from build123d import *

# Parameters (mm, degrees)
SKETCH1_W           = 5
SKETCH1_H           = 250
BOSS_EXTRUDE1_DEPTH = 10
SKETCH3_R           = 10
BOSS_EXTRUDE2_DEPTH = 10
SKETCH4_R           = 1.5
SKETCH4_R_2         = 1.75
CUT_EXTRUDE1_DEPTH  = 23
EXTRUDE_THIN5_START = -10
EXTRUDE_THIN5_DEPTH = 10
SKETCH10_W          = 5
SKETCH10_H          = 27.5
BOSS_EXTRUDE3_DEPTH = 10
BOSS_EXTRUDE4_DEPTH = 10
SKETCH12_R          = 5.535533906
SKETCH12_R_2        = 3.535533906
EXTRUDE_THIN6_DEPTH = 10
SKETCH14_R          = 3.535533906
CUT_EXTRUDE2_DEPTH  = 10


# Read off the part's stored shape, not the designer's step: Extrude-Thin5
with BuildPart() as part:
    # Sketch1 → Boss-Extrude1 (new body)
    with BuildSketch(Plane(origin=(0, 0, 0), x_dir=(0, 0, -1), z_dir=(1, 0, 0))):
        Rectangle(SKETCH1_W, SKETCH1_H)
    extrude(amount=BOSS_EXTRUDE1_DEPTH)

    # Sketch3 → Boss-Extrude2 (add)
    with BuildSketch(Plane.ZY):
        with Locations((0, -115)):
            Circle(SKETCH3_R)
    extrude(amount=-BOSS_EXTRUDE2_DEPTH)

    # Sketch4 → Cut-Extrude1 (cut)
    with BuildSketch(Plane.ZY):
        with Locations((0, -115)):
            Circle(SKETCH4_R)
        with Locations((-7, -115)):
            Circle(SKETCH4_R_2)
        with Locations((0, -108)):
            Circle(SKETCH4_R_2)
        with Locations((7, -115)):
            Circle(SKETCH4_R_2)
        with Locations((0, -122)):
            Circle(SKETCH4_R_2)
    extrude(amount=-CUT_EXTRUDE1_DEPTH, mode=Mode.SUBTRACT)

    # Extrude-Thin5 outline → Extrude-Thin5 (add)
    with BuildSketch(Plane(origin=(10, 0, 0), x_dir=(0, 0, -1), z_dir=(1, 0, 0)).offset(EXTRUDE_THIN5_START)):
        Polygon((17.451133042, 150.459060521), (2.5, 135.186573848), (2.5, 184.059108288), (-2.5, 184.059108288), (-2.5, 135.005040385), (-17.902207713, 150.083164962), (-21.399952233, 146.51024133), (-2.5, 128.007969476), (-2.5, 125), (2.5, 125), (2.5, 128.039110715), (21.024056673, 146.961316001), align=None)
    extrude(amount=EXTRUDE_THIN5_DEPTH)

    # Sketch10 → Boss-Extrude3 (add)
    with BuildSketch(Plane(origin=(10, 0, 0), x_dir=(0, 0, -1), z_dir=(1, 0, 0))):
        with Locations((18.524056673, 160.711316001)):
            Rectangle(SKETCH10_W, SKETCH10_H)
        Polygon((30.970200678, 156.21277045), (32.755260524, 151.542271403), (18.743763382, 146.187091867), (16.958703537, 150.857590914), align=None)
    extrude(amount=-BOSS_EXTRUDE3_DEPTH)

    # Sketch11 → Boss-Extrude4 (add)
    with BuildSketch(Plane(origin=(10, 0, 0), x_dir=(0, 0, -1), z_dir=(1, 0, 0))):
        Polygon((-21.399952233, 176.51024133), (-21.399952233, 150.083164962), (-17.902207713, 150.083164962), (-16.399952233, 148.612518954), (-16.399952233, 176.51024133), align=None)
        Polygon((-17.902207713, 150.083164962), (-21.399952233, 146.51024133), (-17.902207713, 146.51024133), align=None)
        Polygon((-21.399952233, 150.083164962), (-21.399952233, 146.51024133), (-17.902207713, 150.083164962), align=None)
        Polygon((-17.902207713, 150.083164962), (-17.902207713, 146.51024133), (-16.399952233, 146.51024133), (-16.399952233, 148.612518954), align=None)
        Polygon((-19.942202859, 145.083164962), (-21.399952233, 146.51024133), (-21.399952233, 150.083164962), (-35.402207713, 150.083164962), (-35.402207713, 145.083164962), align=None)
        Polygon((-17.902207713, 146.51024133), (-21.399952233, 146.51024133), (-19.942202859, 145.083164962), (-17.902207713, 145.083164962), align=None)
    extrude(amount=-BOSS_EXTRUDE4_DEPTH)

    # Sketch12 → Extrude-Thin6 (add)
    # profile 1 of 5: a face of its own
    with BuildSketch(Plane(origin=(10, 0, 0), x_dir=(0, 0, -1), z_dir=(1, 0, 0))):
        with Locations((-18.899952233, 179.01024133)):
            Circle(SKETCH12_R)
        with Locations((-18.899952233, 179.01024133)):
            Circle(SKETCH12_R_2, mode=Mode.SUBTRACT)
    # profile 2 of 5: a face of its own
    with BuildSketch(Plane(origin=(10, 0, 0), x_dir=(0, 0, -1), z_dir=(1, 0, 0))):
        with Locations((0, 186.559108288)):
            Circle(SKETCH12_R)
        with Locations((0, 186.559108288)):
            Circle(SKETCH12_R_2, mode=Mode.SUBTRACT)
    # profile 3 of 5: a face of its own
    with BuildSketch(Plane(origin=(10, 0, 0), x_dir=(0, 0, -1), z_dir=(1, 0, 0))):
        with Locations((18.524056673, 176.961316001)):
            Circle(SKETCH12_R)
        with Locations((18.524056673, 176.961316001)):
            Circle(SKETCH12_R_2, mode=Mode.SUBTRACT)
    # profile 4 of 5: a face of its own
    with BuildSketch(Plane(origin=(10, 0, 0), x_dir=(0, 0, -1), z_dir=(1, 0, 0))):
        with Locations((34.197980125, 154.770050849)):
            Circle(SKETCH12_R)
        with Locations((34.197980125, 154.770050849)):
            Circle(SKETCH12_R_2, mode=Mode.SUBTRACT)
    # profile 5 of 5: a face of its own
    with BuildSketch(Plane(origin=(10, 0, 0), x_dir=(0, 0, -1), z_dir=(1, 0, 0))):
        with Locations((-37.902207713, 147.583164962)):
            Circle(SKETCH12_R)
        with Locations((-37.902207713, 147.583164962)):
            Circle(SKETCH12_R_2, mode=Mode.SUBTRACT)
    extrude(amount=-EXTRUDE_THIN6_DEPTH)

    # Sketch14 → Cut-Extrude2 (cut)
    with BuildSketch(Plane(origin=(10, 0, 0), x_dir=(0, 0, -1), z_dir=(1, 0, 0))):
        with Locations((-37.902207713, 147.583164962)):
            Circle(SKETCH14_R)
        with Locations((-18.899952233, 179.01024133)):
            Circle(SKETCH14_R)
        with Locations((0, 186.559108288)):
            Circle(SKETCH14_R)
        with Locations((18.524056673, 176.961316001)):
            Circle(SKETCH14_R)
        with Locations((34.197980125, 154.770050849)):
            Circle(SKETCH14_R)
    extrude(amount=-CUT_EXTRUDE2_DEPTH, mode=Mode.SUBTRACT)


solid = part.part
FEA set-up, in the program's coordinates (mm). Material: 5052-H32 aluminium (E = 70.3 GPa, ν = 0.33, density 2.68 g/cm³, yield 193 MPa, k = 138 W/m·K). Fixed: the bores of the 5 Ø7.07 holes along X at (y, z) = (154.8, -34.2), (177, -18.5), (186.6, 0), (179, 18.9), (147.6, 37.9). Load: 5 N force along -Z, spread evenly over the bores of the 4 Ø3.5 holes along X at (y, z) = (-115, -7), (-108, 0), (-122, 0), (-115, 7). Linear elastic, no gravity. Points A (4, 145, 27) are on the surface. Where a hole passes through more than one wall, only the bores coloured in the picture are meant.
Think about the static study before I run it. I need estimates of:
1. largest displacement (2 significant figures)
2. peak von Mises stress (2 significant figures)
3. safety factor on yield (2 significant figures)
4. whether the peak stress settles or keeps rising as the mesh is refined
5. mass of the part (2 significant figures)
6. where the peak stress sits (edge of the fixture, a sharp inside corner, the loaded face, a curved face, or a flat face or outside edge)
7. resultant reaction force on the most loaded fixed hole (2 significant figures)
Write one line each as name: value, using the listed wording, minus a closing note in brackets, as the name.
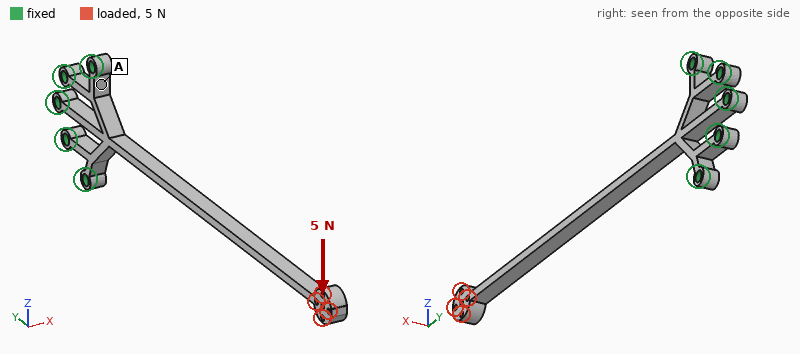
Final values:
largest displacement: 3.6 mm
peak von Mises stress: 28 MPa
safety factor on yield: 6.9
whether the peak stress settles or keeps rising as the mesh is refined: settles
mass of the part: 69 g
where the peak stress sits: a flat face or outside edge
resultant reaction force on the most loaded fixed hole: 44 N
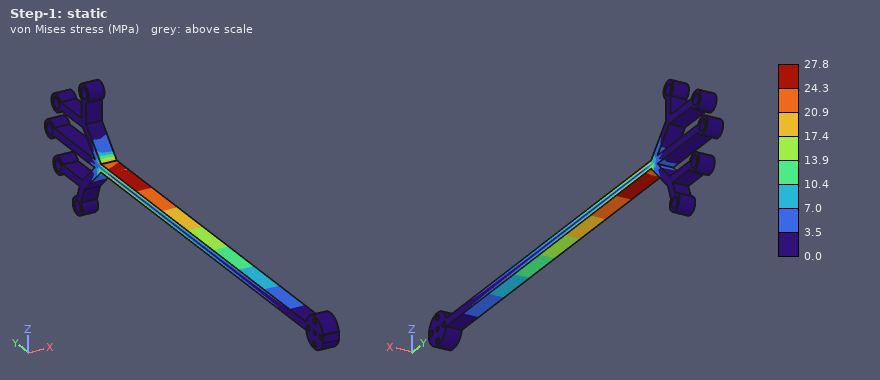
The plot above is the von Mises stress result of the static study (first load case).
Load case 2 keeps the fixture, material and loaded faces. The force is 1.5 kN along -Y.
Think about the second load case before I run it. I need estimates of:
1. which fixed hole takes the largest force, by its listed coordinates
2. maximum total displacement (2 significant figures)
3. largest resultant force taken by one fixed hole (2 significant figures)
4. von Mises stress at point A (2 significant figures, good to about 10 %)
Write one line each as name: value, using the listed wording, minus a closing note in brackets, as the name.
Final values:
which fixed hole takes the largest force, by its listed coordinates: (186.6, 0)
maximum total displacement: 0.11 mm
largest resultant force taken by one fixed hole: 630 N
von Mises stress at point A: 5.1 MPa
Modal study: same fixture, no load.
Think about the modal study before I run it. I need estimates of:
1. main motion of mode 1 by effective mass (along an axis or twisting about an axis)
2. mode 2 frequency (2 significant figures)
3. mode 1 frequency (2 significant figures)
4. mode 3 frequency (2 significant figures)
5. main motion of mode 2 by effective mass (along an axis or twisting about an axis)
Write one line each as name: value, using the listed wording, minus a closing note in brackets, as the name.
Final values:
main motion of mode 1 by effective mass: along Z
mode 2 frequency: 94 Hz
mode 1 frequency: 52 Hz
mode 3 frequency: 350 Hz
main motion of mode 2 by effective mass: along X
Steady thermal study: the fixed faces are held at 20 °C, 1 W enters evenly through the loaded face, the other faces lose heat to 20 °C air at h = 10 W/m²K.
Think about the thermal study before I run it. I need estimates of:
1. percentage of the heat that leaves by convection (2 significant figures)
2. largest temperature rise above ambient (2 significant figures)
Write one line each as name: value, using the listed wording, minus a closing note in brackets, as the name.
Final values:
percentage of the heat that leaves by convection: 71 %
largest temperature rise above ambient: 17 K
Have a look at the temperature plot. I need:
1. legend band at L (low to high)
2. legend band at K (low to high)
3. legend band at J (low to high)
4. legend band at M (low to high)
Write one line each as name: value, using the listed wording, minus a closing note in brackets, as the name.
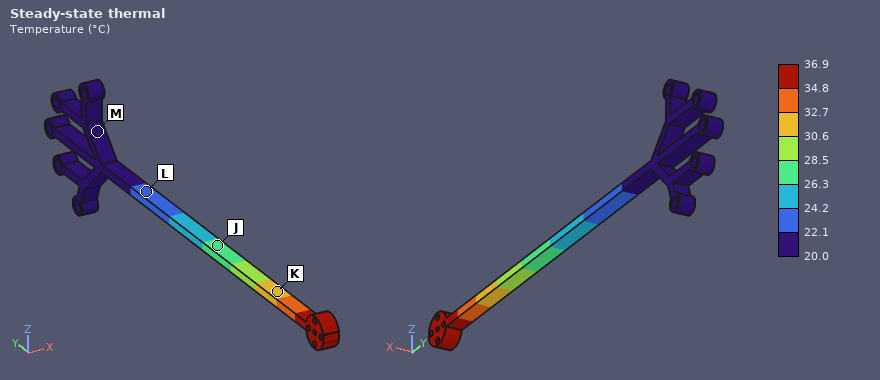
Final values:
legend band at L: 22.1 to 24.2 °C
legend band at K: 30.6 to 32.7 °C
legend band at J: 26.3 to 28.5 °C
legend band at M: 20.0 to 22.1 °C
